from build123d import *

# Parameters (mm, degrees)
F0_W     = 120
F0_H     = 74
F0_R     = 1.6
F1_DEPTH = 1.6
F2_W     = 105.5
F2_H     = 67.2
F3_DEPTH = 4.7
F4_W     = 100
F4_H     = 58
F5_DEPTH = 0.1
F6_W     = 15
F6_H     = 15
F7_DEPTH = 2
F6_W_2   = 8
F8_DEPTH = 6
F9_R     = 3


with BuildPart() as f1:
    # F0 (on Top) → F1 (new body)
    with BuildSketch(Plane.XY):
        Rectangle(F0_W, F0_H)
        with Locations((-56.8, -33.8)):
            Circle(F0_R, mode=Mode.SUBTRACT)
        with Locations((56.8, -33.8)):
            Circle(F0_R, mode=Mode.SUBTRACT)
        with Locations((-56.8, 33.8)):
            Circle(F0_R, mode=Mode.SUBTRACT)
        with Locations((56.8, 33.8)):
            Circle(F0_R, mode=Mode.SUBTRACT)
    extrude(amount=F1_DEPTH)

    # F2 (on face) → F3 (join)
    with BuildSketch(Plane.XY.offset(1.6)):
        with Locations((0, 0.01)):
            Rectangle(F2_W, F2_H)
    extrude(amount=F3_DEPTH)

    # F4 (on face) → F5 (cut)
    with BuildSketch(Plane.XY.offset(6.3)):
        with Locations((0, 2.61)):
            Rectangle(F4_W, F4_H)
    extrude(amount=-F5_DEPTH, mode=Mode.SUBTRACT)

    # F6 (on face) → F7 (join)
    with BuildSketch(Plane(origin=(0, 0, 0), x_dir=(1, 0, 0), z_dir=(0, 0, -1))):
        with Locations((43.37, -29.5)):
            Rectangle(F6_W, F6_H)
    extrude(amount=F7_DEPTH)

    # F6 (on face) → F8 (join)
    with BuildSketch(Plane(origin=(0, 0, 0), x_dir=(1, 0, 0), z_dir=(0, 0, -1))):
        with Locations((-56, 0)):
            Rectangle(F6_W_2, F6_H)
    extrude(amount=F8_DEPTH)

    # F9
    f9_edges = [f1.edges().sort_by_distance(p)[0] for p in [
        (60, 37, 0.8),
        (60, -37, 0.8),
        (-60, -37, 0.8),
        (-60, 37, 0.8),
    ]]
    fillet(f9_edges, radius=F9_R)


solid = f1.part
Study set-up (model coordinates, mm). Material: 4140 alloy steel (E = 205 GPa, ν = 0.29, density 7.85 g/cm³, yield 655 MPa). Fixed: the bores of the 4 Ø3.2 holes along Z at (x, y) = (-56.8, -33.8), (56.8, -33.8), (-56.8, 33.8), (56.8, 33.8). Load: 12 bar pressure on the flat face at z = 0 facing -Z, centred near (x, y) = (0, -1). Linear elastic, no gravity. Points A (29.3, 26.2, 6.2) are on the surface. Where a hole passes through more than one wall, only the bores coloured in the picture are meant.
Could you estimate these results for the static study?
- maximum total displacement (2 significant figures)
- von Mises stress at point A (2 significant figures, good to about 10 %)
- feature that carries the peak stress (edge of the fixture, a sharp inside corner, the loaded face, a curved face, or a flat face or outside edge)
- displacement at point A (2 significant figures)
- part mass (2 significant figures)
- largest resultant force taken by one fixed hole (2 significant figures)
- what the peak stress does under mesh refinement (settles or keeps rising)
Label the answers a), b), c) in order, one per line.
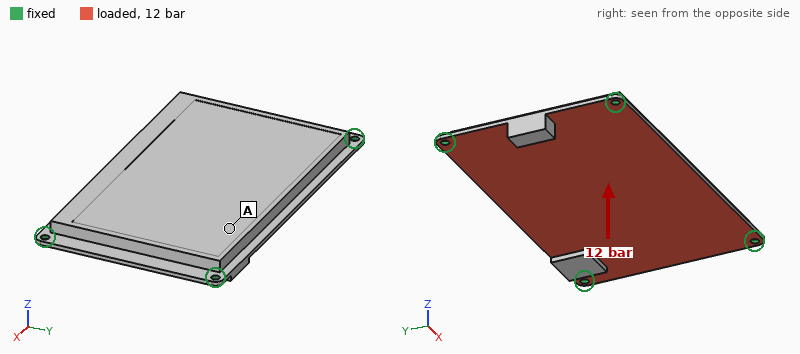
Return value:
a) 0.47 mm
b) 190 MPa
c) edge of the fixture
d) 0.31 mm
e) 380 g
f) 7.4 kN
g) keeps rising
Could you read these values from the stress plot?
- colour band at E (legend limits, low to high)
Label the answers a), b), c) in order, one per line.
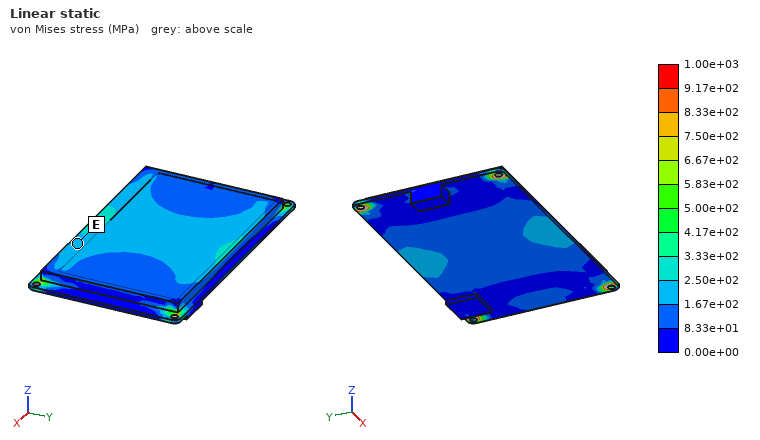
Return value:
a) 1.67e+02 to 2.50e+02 MPa
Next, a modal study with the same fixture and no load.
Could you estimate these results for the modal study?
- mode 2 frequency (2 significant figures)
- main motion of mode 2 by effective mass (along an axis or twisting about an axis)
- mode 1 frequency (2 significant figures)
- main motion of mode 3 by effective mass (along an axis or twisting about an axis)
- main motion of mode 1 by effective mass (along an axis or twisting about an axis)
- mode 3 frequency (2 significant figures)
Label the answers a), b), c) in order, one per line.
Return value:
a) 2700 Hz
b) twisting about X
c) 1400 Hz
d) twisting about Y
e) along Z
f) 3300 Hz
